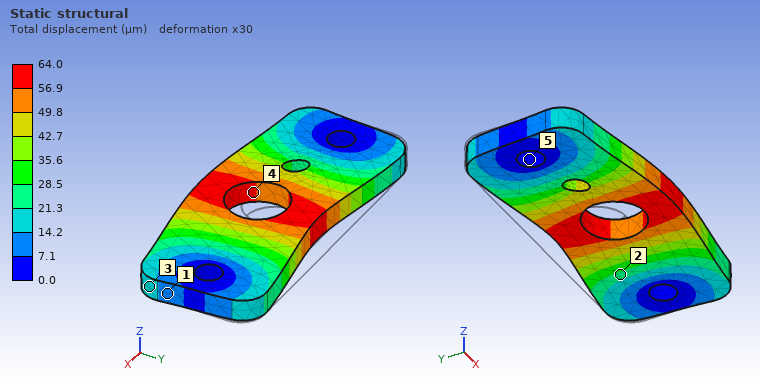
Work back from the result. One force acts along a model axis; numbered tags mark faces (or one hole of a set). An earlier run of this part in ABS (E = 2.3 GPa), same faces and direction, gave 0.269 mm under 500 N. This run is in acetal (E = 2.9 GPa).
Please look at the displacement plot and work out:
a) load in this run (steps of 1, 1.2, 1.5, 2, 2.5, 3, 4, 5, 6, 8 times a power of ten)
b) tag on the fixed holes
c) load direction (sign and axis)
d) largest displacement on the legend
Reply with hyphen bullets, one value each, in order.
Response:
- 150 N
- 5
- -Y
- 64.0 µm
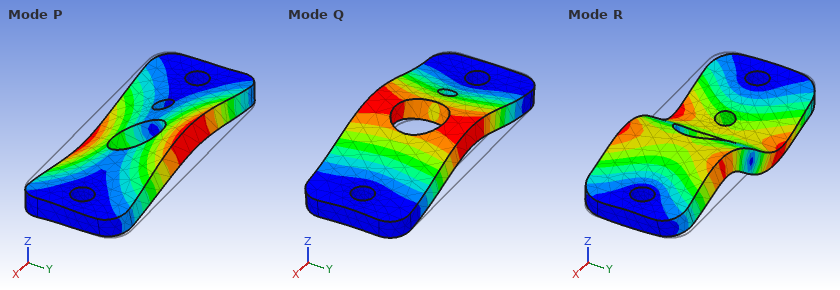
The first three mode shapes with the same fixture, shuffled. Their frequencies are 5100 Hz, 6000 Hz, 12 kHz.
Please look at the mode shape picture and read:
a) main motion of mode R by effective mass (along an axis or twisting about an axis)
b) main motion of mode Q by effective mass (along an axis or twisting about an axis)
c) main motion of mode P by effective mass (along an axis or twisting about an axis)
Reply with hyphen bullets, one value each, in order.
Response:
- twisting about Y
- along Z
- twisting about X
